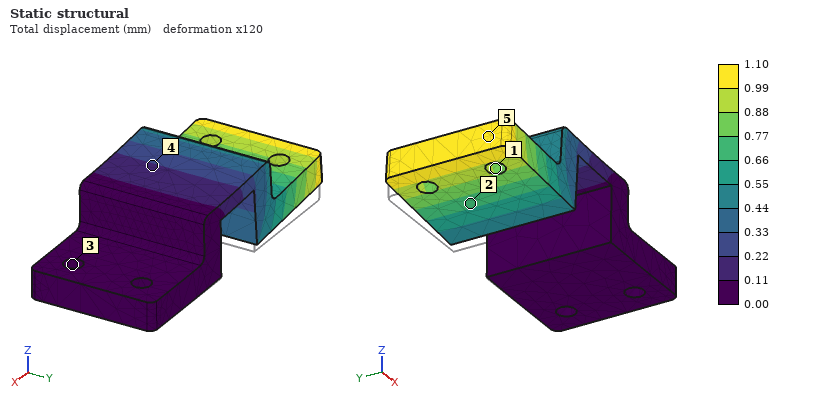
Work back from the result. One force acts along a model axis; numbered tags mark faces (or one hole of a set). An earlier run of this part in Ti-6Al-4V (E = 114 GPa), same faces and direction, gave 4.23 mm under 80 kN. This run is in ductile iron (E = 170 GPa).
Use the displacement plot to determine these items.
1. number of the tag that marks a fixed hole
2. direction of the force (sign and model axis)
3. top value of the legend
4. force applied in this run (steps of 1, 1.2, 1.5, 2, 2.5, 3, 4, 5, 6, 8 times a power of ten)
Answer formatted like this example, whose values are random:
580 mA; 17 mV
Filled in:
3; +Z; 1.10 mm; 30 kN
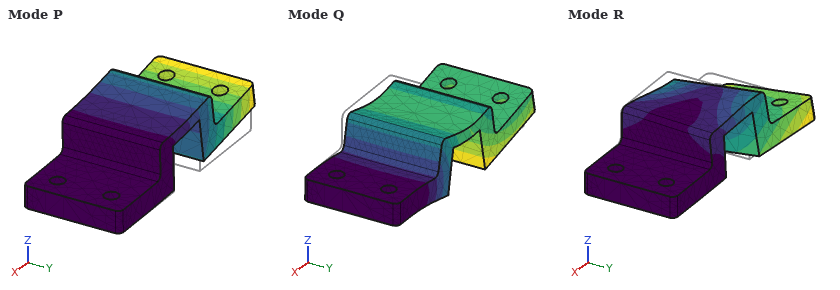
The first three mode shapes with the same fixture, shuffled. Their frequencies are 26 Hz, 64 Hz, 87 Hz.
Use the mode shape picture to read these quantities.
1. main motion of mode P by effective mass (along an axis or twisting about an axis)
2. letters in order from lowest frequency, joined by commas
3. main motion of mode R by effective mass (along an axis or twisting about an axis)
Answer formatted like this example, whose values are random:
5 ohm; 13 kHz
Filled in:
along Z; P, R, Q; along Y
